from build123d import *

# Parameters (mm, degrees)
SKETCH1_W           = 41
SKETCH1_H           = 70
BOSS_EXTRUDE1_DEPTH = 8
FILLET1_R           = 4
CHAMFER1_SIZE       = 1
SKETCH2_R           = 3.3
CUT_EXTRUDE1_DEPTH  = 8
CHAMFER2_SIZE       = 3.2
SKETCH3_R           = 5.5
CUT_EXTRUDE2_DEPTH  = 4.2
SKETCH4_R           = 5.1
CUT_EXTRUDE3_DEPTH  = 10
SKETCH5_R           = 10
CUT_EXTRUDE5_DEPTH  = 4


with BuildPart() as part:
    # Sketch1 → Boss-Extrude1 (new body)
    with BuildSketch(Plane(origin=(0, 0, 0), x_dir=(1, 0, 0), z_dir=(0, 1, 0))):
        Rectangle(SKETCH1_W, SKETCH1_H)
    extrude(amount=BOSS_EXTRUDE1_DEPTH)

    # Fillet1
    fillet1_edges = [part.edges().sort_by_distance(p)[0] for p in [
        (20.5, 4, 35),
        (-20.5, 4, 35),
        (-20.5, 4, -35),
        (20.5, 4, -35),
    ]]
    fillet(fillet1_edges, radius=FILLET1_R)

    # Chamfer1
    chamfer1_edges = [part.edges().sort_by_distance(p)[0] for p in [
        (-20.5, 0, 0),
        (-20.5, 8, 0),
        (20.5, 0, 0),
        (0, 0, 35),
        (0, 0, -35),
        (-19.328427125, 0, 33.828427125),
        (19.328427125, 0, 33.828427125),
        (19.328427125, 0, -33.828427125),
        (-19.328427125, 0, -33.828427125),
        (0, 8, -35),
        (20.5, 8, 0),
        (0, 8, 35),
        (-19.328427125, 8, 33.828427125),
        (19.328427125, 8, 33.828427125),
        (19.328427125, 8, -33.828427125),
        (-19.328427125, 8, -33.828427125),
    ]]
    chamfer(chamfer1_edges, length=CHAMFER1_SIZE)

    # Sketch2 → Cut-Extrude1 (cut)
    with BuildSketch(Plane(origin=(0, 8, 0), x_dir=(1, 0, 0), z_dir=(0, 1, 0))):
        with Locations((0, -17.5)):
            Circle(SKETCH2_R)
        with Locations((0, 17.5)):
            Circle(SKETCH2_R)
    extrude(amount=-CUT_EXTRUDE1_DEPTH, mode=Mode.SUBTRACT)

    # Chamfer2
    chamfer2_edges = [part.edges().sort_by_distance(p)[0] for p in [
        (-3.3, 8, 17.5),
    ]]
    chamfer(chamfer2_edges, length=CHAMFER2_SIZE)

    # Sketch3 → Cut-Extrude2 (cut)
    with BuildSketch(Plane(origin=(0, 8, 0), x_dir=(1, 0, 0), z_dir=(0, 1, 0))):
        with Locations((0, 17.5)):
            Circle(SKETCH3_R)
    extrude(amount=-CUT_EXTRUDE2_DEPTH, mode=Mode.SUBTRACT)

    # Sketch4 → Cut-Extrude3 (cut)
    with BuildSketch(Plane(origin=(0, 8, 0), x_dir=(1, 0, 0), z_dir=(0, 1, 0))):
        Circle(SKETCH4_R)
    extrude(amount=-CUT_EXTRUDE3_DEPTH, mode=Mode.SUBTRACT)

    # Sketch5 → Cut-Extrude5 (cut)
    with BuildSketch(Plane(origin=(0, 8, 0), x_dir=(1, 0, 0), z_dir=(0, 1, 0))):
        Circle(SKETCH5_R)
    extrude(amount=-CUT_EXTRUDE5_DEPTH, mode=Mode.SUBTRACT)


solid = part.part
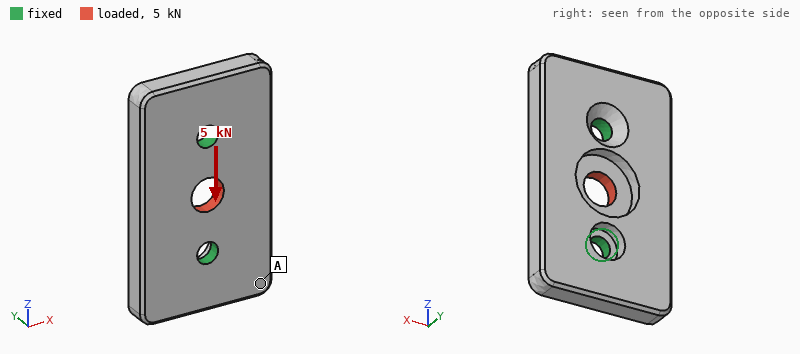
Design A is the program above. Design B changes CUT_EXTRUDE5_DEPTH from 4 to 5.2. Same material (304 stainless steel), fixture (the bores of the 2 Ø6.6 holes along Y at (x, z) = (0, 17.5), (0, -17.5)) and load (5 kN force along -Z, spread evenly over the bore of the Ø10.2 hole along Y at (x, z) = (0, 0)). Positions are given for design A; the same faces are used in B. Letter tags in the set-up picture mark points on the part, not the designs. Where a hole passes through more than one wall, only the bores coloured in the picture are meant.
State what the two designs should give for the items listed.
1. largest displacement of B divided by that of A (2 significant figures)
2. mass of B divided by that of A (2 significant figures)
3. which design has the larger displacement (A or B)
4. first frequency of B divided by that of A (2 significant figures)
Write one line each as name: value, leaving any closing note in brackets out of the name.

largest displacement of B divided by that of A: 1.3
mass of B divided by that of A: 0.99
which design has the larger displacement: B
first frequency of B divided by that of A: 0.99
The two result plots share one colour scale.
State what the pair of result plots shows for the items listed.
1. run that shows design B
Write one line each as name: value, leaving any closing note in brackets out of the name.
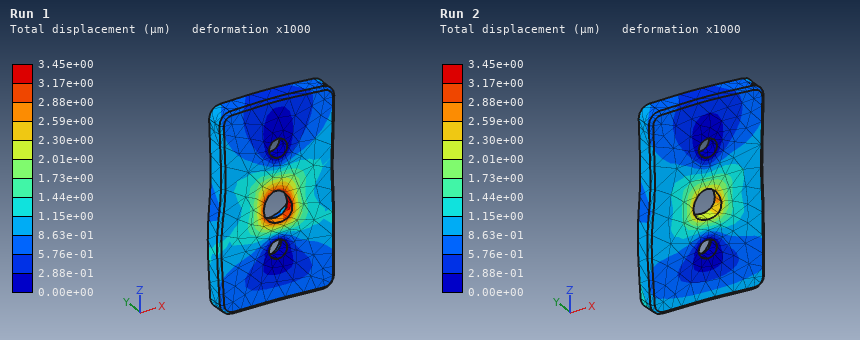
run that shows design B: Run 1
